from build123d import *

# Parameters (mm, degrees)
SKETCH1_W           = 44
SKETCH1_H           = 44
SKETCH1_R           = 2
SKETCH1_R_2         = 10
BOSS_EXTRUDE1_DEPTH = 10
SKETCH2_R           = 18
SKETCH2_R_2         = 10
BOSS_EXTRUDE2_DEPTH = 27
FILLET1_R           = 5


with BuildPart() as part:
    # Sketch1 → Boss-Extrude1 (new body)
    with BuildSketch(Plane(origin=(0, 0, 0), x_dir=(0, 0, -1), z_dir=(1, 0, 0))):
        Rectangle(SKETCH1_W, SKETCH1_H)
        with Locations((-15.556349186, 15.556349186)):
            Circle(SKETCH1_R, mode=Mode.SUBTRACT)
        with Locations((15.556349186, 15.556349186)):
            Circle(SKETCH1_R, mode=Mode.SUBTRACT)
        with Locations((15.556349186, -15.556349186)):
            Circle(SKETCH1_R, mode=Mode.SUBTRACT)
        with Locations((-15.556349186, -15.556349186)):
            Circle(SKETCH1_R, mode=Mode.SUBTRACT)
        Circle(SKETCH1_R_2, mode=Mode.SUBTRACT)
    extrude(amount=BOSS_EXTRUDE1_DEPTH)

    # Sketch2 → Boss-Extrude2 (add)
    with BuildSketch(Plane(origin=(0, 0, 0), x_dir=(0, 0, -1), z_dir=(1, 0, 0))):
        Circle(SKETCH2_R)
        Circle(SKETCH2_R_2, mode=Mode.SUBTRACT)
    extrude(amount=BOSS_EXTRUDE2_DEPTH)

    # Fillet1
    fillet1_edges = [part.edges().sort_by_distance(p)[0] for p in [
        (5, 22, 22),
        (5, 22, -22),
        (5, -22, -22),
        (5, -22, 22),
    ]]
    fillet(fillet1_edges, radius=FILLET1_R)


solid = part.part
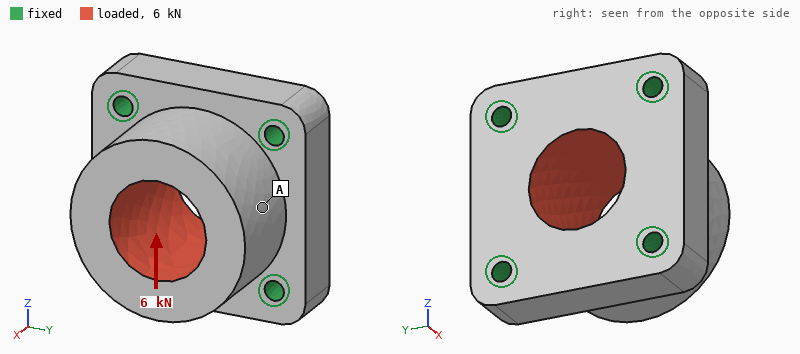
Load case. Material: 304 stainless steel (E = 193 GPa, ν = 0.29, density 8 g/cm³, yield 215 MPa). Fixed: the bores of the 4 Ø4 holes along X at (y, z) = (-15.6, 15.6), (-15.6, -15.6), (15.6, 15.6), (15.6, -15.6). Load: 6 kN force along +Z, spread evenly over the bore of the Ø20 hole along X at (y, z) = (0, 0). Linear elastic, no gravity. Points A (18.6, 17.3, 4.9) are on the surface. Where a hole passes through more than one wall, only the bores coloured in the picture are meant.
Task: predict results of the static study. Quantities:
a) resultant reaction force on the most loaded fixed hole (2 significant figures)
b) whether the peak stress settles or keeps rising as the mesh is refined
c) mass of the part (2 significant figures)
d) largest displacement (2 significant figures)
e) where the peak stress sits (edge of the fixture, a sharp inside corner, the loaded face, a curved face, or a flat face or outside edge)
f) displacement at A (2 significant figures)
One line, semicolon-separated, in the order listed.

1.7 kN; keeps rising; 220 g; 3.3 µm; edge of the fixture; 1.9 µm
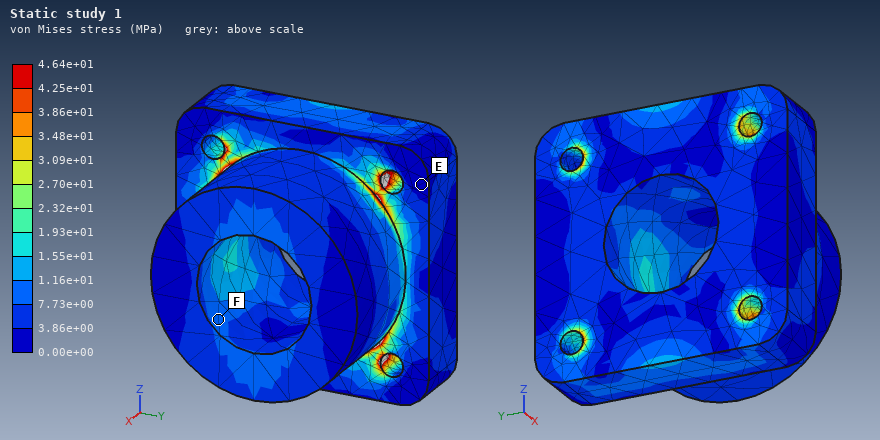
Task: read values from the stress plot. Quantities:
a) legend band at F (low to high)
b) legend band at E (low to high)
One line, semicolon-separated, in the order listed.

7.73e+00 to 1.16e+01 MPa; 0.00e+00 to 3.86e+00 MPa
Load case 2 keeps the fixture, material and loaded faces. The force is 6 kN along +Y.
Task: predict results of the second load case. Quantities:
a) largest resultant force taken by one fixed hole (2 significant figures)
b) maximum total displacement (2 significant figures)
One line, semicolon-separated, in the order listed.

1.7 kN; 3.3 µm
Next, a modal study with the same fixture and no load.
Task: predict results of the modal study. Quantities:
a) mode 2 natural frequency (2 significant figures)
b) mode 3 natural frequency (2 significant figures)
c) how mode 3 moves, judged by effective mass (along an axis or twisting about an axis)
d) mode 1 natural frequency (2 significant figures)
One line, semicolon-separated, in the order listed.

20 kHz; 25 kHz; along X; 20 kHz
